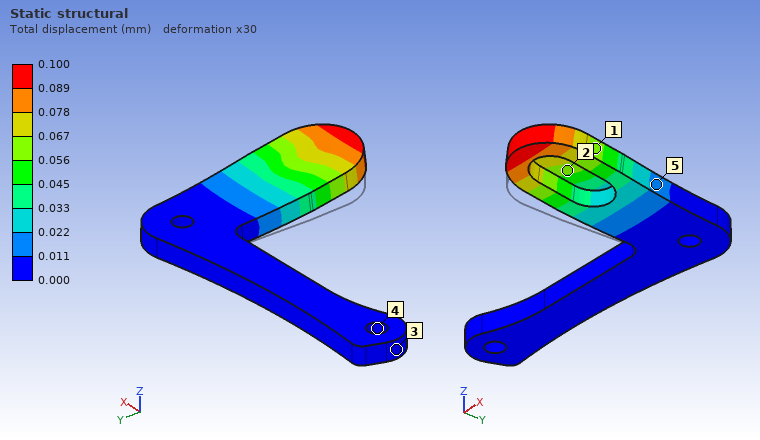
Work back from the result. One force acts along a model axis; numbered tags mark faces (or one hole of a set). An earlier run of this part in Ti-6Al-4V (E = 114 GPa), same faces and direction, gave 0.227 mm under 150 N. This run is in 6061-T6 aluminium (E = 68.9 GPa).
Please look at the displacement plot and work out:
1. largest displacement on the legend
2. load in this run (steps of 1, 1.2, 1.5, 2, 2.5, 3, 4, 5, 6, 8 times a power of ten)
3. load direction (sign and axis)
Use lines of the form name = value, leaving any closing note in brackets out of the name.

largest displacement on the legend = 0.100 mm
load in this run = 40 N
load direction = +Z
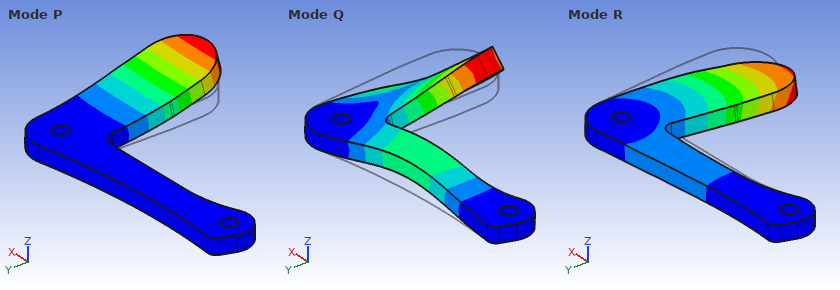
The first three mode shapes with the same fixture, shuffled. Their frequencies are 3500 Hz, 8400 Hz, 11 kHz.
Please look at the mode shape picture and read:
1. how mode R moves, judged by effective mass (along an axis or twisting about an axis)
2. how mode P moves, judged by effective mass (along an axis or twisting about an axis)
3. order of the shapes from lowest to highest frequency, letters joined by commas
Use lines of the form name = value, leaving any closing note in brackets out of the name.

how mode R moves, judged by effective mass = along X
how mode P moves, judged by effective mass = along Z
order of the shapes from lowest to highest frequency, letters joined by commas = P, R, Q
